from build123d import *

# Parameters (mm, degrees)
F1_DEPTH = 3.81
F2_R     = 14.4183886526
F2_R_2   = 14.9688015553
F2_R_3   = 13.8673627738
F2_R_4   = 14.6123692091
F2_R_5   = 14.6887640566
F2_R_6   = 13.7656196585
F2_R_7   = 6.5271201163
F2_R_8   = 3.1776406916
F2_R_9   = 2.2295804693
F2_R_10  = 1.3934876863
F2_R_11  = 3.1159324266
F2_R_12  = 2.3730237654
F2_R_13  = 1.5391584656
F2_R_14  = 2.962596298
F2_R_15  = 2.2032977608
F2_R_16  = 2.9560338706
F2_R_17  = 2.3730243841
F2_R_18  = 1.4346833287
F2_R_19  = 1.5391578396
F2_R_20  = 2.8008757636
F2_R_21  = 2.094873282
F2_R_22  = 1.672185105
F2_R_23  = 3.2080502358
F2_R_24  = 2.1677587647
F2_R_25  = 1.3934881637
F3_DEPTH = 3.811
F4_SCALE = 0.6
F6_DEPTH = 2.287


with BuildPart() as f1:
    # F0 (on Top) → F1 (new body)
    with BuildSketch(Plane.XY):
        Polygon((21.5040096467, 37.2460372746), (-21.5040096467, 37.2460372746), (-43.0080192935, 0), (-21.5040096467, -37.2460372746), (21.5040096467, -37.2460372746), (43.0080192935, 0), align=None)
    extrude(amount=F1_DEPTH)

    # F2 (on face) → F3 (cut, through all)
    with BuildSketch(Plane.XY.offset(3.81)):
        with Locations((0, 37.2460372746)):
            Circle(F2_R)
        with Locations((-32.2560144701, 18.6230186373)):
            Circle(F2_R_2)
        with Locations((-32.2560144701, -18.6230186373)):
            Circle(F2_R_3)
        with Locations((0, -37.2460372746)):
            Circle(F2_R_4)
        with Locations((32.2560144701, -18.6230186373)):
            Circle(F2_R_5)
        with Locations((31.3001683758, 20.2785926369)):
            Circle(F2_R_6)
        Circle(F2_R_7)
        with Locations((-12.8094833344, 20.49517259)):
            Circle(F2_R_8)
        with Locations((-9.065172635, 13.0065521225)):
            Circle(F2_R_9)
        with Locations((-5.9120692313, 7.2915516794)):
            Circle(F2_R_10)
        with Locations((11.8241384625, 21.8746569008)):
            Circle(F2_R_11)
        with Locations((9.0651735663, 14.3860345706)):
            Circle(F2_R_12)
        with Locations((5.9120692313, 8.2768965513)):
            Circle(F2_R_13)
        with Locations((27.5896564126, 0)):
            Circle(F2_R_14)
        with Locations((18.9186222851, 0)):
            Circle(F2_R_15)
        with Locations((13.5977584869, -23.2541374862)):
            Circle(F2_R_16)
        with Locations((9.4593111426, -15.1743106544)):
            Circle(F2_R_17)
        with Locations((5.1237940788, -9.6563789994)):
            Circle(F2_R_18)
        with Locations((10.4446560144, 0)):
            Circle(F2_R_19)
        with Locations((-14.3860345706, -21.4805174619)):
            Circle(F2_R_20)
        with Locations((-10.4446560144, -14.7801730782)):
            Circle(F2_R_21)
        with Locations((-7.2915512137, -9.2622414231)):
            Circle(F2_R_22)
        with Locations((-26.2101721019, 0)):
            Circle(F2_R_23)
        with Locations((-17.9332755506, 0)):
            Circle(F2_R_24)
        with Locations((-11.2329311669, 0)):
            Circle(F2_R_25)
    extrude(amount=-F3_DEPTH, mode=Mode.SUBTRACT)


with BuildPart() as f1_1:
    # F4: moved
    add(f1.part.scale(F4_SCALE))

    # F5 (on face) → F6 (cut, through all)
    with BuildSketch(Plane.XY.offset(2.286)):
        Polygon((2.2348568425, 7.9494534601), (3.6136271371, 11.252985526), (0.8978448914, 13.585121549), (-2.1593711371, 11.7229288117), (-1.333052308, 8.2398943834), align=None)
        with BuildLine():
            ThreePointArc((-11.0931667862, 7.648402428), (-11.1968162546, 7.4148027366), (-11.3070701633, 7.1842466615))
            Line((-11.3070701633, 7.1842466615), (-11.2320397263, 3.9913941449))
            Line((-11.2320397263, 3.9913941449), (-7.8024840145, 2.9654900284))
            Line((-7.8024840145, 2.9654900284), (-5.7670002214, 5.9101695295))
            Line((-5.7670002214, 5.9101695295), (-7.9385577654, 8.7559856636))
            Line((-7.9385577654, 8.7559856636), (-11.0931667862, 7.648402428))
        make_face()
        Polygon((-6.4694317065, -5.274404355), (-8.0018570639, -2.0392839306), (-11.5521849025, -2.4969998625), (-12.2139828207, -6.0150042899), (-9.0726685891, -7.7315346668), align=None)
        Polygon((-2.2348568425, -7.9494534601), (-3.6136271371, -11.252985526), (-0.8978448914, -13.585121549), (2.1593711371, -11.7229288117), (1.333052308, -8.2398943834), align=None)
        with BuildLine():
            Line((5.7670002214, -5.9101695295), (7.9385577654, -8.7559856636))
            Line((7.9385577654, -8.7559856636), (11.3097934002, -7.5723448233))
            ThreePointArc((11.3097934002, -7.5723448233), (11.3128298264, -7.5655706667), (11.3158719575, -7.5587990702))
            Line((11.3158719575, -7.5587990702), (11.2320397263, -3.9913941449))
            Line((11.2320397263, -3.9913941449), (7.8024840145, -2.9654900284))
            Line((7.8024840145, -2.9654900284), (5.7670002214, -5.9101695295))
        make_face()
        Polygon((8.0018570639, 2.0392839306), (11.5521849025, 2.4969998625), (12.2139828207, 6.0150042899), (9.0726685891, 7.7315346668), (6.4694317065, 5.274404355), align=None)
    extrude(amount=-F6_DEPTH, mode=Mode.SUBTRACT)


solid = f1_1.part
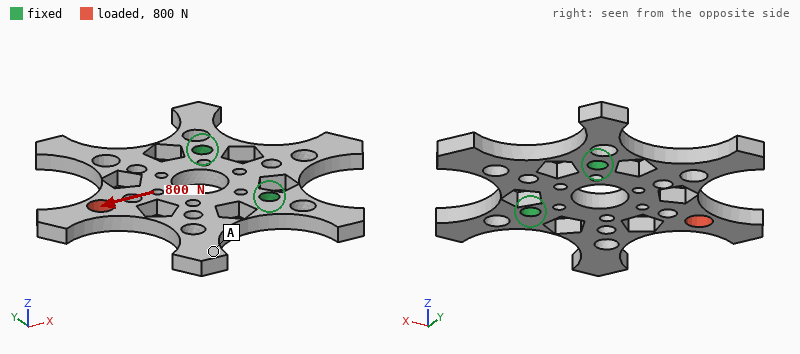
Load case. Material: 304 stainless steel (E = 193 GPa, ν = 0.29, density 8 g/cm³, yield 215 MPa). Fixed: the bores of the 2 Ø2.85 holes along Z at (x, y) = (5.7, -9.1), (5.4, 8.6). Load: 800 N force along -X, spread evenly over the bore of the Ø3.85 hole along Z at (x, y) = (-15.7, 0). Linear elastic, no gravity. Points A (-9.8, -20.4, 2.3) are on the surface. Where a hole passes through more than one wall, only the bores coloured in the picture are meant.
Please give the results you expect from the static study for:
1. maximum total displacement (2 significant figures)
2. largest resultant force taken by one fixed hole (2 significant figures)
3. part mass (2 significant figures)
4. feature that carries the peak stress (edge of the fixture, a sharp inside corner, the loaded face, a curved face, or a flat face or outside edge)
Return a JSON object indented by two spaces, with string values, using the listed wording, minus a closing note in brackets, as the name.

{
  "maximum total displacement": "12 µm",
  "largest resultant force taken by one fixed hole": "450 N",
  "part mass": "13 g",
  "feature that carries the peak stress": "a curved face"
}
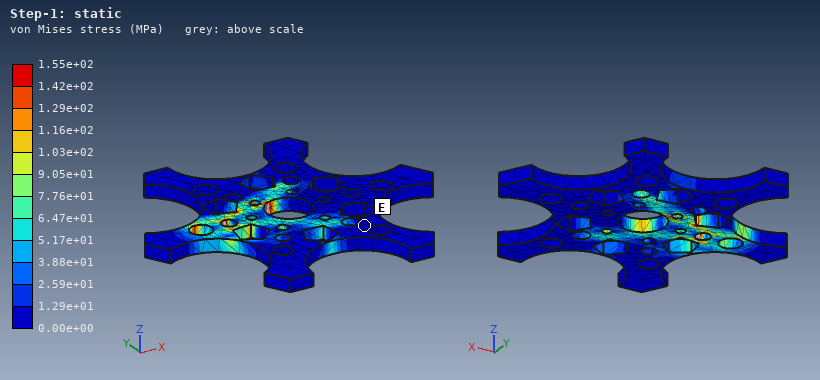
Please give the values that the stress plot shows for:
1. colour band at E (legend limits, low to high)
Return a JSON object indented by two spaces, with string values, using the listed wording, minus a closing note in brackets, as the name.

{
  "colour band at E": "0.00e+00 to 1.29e+01 MPa"
}
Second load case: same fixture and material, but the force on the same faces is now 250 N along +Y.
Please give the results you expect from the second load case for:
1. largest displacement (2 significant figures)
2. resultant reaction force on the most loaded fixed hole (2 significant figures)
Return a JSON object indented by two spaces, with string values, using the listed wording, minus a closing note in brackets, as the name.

{
  "largest displacement": "20 µm",
  "resultant reaction force on the most loaded fixed hole": "310 N"
}
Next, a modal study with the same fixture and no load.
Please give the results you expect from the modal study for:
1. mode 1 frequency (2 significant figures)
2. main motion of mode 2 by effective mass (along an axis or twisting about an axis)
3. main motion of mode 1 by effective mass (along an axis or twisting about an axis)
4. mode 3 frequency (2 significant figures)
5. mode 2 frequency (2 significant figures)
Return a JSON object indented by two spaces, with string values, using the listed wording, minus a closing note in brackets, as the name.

{
  "mode 1 frequency": "2200 Hz",
  "main motion of mode 2 by effective mass": "twisting about X",
  "main motion of mode 1 by effective mass": "along Z",
  "mode 3 frequency": "4100 Hz",
  "mode 2 frequency": "3500 Hz"
}
